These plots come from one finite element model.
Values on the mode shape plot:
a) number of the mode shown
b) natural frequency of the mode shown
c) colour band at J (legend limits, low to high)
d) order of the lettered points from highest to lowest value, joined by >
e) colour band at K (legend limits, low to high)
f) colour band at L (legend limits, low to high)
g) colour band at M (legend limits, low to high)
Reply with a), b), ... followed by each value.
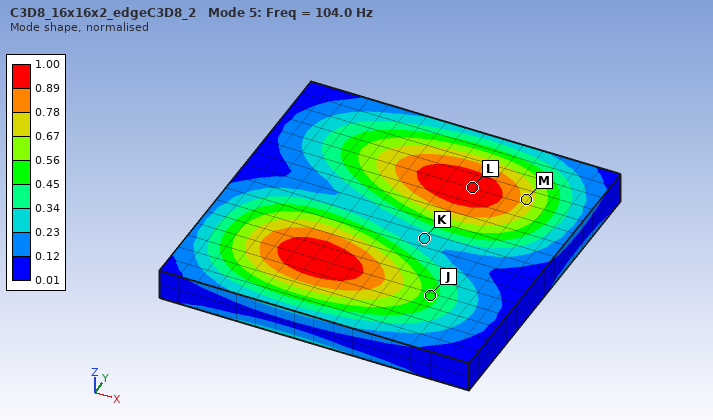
a) 5
b) 104.0 Hz
c) 0.45 to 0.56
d) L > M > J > K
e) 0.23 to 0.34
f) 0.89 to 1.00
g) 0.67 to 0.78
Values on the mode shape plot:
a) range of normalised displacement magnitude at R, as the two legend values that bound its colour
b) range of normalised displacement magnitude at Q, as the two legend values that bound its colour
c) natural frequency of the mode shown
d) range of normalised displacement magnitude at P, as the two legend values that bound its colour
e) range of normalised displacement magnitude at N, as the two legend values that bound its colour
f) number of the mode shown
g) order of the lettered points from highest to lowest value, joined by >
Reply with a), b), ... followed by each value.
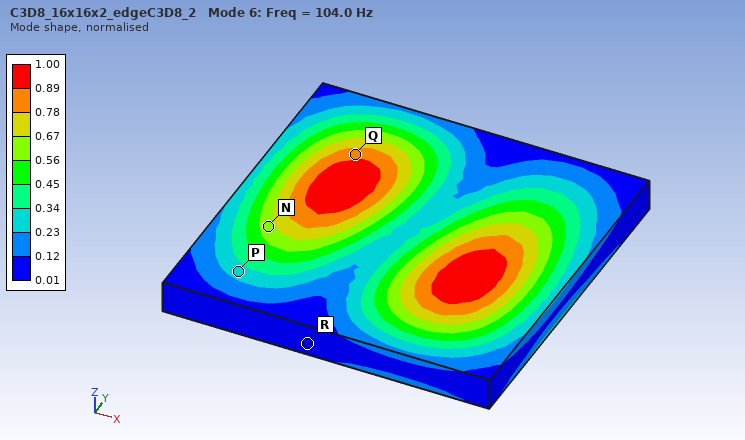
a) 0.01 to 0.12
b) 0.78 to 0.89
c) 104.0 Hz
d) 0.23 to 0.34
e) 0.56 to 0.67
f) 6
g) Q > N > P > R
